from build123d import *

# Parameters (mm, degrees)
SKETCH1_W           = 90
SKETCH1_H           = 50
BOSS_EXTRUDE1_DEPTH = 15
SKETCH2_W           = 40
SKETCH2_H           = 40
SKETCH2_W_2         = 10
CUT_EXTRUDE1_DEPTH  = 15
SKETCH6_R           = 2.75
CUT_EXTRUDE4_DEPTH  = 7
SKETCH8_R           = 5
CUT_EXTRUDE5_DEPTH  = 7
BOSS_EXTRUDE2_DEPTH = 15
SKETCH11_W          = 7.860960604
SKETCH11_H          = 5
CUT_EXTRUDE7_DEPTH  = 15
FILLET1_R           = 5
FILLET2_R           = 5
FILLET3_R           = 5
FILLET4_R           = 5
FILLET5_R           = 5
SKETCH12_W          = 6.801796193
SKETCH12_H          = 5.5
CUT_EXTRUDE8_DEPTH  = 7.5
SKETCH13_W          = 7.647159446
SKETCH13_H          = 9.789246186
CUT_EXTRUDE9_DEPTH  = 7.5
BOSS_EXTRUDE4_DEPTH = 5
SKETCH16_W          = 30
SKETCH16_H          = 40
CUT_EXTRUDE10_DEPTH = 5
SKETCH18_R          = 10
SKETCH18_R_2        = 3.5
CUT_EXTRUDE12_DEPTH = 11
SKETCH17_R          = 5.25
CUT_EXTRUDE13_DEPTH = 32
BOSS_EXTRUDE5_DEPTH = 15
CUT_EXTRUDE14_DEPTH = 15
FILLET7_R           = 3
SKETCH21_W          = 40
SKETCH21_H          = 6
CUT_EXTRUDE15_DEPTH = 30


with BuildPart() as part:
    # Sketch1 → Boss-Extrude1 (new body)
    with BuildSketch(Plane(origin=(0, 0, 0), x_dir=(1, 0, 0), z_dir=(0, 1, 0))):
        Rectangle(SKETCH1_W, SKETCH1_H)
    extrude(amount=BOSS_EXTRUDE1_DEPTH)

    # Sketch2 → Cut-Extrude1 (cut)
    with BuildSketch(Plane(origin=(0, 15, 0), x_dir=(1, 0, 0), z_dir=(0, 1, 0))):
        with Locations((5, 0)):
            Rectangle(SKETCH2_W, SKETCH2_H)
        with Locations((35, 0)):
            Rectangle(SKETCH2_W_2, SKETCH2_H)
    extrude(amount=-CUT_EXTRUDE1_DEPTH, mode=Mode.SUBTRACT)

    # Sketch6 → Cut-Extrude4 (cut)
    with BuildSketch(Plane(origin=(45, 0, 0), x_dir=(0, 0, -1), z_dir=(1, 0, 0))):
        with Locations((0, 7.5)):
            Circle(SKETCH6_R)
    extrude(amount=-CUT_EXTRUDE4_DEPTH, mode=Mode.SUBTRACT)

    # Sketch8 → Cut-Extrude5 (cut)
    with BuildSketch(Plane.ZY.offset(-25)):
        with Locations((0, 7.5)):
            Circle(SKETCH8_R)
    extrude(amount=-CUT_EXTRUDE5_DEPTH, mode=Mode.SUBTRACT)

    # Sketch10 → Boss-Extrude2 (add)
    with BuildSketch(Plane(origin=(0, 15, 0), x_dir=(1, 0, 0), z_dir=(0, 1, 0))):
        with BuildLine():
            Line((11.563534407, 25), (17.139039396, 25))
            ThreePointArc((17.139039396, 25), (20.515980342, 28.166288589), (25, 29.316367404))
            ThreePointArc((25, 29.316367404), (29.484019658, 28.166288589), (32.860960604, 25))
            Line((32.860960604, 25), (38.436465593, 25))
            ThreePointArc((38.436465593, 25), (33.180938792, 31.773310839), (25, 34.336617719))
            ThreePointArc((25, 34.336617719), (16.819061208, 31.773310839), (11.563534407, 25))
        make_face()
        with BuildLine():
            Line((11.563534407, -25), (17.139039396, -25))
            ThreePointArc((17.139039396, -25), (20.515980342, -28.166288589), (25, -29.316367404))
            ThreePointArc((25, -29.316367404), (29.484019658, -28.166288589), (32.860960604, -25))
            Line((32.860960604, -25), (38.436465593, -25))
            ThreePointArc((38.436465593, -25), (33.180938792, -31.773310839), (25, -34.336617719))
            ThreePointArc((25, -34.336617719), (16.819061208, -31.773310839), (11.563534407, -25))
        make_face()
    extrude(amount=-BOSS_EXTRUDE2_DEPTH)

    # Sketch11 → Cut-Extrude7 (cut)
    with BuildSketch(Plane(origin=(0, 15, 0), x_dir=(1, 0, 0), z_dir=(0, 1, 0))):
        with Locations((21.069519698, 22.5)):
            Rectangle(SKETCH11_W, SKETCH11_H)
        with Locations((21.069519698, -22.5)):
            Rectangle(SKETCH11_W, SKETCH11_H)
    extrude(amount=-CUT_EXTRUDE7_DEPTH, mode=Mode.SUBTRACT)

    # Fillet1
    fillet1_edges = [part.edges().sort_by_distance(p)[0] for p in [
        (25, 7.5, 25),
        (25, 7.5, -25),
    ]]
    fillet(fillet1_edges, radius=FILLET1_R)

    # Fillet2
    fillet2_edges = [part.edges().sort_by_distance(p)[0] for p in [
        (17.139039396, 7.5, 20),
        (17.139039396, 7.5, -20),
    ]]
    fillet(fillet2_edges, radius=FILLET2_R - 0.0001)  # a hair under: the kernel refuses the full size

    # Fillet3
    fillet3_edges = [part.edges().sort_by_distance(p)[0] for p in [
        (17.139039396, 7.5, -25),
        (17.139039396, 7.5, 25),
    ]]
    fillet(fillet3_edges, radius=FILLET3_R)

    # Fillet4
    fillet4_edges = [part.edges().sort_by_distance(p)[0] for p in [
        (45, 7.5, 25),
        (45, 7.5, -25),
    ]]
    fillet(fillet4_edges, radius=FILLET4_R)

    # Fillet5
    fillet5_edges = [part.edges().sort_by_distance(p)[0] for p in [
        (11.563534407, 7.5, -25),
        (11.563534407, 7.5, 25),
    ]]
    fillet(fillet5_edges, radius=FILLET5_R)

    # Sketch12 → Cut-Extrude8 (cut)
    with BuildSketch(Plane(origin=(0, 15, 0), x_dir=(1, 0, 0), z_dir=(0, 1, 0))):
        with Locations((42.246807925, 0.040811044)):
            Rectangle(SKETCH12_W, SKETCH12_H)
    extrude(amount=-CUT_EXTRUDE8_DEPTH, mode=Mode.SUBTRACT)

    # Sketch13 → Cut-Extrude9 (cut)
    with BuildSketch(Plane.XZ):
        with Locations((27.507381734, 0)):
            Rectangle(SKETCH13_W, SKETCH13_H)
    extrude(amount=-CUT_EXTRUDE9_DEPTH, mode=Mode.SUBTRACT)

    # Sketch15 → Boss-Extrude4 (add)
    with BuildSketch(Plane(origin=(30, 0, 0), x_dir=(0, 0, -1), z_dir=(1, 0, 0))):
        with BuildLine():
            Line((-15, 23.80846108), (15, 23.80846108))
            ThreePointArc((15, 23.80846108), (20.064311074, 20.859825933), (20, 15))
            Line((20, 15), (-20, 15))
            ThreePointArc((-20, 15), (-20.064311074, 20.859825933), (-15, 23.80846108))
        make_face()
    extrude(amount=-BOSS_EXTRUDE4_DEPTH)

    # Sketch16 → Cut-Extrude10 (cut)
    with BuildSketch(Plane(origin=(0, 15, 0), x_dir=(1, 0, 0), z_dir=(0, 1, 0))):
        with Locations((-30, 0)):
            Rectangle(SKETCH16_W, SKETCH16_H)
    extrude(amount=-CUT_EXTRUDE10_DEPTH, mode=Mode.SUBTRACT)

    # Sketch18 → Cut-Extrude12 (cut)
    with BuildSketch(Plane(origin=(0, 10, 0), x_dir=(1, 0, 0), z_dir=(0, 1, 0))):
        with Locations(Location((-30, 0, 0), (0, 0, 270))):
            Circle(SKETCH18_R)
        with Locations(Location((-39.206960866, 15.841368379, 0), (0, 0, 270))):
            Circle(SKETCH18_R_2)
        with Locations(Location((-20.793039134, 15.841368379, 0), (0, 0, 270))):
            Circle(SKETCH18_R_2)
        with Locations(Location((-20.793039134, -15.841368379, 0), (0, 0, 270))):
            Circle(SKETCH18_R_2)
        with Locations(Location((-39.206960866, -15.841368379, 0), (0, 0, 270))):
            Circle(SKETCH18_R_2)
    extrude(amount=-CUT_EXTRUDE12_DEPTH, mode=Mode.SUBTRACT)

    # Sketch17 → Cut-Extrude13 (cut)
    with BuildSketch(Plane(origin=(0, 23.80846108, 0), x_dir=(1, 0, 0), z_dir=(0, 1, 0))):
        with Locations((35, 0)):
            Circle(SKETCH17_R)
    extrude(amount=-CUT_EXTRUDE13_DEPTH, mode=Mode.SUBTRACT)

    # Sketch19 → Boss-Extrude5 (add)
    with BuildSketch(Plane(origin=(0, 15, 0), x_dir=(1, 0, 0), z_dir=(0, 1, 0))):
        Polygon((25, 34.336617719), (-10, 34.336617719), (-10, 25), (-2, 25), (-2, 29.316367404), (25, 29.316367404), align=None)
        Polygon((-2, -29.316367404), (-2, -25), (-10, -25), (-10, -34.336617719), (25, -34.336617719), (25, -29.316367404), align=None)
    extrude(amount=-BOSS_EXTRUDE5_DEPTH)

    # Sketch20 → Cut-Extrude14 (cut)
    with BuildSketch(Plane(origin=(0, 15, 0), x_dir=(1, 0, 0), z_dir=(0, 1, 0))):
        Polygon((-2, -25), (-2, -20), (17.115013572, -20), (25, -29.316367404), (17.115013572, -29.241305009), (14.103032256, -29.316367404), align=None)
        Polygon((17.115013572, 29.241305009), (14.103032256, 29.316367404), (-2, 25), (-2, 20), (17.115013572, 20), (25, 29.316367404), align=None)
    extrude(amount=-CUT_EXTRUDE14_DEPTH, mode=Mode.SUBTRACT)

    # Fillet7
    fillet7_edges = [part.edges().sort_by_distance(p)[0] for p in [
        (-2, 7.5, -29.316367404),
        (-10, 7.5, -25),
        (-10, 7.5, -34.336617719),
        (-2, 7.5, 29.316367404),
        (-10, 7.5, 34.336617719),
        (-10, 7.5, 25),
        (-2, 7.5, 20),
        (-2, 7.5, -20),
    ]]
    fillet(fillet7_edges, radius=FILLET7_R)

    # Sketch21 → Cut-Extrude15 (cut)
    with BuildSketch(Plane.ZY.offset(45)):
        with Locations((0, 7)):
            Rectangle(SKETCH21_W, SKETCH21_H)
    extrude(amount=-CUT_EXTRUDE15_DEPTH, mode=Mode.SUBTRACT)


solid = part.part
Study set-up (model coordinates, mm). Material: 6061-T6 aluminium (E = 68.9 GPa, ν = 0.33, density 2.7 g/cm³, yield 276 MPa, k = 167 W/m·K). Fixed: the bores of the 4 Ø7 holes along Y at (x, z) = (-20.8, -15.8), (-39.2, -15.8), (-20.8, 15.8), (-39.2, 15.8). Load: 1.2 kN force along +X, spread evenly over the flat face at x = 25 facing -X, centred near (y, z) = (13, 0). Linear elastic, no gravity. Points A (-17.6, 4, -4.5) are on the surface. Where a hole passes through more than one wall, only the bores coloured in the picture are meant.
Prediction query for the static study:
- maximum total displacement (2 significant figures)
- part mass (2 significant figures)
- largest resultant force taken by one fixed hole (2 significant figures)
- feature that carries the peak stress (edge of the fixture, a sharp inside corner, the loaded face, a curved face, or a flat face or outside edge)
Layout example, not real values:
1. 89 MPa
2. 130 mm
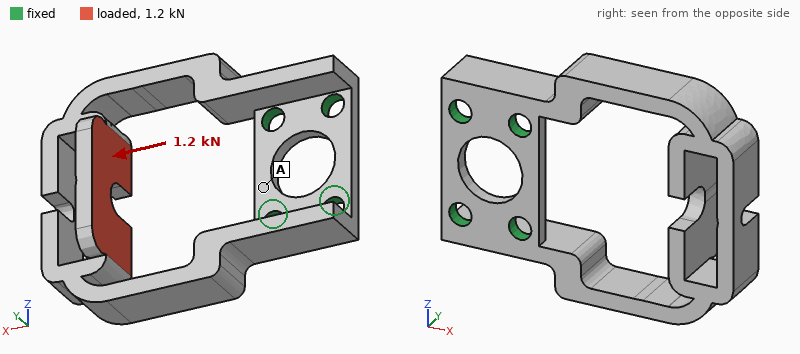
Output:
1. 0.20 mm
2. 74 g
3. 530 N
4. the loaded face
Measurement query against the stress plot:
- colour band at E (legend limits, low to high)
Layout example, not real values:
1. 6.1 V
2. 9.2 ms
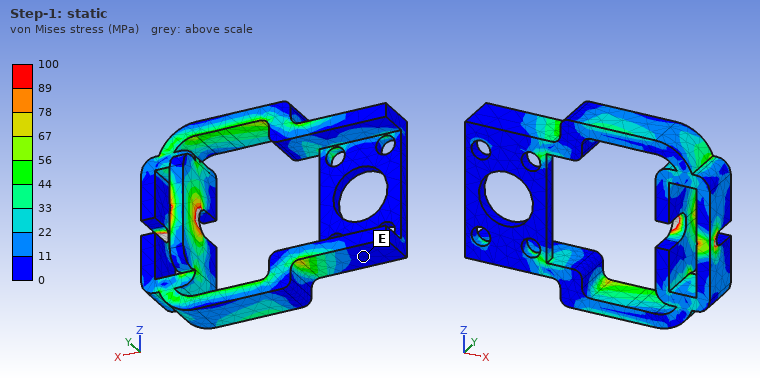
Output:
1. 0 to 11 MPa
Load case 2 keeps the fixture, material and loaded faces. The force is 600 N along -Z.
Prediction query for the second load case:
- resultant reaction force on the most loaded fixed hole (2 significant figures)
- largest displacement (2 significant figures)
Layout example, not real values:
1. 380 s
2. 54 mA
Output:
1. 730 N
2. 0.63 mm
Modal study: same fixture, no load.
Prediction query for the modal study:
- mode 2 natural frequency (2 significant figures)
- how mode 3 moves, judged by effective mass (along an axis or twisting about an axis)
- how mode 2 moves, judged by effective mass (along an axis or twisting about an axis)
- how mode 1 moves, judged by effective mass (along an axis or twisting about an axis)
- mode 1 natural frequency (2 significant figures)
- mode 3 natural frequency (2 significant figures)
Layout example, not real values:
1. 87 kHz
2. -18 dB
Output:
1. 1200 Hz
2. twisting about X
3. along Y
4. along Z
5. 840 Hz
6. 2100 Hz
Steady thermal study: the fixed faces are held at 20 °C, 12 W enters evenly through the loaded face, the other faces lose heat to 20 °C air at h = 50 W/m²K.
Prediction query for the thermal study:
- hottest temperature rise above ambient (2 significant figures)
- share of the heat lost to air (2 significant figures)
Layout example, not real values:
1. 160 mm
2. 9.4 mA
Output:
1. 23 K
2. 50 %
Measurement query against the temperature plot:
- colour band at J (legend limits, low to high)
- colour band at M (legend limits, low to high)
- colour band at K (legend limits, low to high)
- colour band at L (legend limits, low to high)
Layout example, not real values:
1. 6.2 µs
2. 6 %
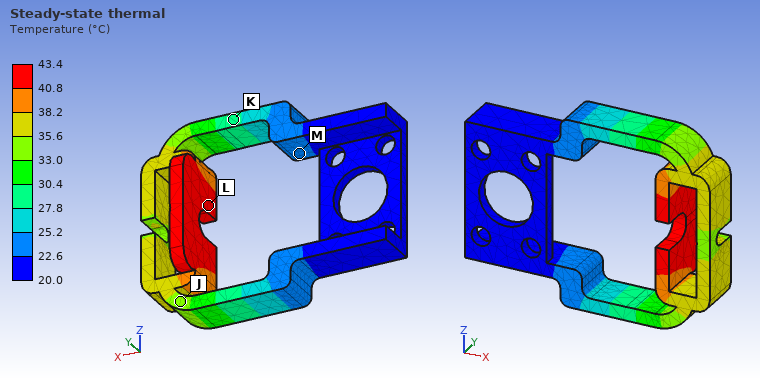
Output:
1. 33.0 to 35.6 °C
2. 22.6 to 25.2 °C
3. 27.8 to 30.4 °C
4. 40.8 to 43.4 °C
